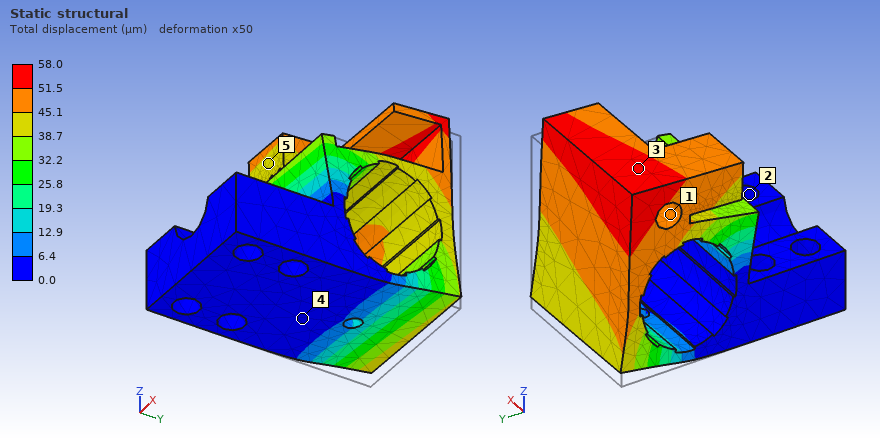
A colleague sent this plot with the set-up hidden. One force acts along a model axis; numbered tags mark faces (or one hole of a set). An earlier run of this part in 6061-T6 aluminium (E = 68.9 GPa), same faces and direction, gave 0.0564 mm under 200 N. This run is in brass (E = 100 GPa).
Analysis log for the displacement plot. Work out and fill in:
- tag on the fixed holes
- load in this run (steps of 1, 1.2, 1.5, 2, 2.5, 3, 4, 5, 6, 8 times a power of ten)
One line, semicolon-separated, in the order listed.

2; 300 N
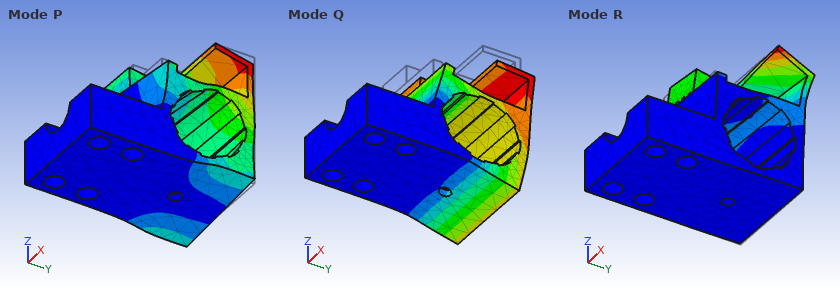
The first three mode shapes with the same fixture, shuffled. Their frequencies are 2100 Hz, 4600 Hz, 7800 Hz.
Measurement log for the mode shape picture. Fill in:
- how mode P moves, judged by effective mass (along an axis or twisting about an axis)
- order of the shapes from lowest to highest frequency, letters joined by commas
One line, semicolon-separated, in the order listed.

along X; Q, P, R
